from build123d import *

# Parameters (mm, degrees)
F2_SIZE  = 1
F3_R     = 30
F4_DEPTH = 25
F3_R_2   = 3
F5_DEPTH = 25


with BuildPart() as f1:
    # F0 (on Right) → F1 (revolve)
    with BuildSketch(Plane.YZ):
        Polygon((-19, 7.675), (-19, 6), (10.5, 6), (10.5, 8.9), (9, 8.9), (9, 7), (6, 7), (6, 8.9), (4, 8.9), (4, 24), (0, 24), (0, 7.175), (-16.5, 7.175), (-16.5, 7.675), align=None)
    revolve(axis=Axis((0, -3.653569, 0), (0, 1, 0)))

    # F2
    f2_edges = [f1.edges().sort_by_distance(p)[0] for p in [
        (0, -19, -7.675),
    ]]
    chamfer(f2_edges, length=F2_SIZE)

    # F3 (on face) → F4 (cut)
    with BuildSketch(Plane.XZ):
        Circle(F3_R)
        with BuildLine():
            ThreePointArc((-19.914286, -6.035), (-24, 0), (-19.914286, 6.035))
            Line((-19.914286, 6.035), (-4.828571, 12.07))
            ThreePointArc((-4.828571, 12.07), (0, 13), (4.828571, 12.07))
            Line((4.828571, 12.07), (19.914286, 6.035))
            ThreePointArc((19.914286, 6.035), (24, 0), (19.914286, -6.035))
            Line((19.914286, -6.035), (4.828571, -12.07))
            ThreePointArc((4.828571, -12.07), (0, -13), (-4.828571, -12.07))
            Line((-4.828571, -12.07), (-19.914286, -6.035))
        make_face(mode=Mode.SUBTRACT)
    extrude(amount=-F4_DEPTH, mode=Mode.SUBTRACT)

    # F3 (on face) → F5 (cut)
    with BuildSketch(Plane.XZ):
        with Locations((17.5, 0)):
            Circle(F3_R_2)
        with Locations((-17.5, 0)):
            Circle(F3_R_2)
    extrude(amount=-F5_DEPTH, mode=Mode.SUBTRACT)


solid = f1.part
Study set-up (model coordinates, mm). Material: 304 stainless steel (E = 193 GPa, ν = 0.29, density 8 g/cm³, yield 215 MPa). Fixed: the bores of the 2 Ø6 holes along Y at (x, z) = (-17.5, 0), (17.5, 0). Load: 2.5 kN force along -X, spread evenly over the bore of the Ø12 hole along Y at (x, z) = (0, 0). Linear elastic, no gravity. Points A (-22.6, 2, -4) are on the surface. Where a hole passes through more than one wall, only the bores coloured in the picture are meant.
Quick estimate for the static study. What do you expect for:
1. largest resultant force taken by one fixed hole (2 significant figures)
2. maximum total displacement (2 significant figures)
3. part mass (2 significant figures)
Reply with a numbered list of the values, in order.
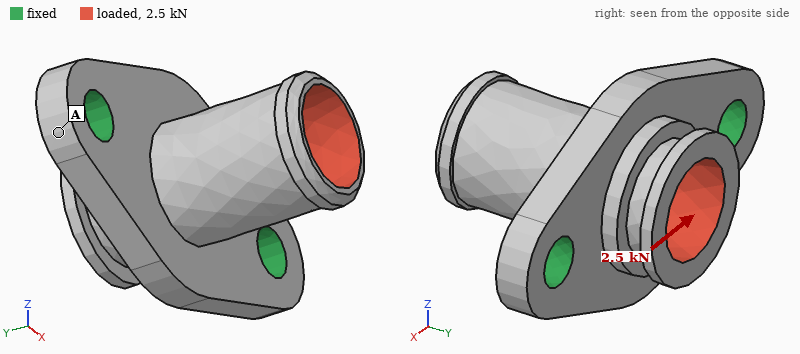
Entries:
1. 1.4 kN
2. 31 µm
3. 35 g
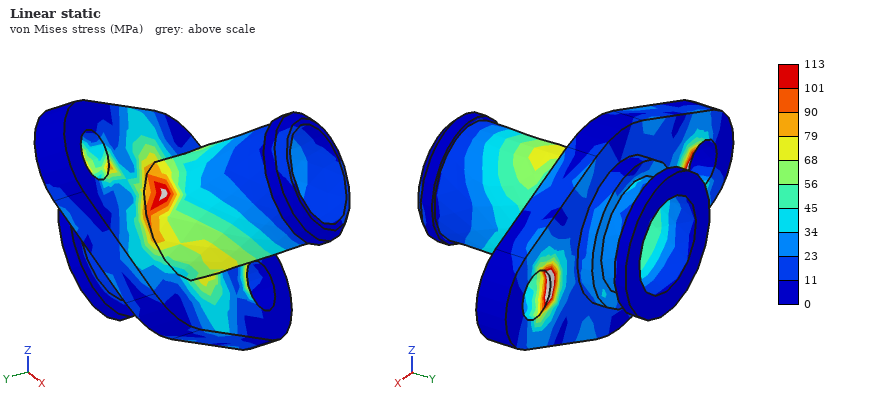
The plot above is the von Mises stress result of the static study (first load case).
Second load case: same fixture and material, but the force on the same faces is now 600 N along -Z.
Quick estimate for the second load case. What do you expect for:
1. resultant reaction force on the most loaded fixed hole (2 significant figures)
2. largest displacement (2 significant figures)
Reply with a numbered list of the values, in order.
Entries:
1. 300 N
2. 18 µm
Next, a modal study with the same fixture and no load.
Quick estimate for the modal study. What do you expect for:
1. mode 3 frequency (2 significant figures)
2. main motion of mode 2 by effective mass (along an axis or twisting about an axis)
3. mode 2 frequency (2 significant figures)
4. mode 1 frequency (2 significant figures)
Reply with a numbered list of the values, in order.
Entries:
1. 14 kHz
2. along Y
3. 14 kHz
4. 7800 Hz
